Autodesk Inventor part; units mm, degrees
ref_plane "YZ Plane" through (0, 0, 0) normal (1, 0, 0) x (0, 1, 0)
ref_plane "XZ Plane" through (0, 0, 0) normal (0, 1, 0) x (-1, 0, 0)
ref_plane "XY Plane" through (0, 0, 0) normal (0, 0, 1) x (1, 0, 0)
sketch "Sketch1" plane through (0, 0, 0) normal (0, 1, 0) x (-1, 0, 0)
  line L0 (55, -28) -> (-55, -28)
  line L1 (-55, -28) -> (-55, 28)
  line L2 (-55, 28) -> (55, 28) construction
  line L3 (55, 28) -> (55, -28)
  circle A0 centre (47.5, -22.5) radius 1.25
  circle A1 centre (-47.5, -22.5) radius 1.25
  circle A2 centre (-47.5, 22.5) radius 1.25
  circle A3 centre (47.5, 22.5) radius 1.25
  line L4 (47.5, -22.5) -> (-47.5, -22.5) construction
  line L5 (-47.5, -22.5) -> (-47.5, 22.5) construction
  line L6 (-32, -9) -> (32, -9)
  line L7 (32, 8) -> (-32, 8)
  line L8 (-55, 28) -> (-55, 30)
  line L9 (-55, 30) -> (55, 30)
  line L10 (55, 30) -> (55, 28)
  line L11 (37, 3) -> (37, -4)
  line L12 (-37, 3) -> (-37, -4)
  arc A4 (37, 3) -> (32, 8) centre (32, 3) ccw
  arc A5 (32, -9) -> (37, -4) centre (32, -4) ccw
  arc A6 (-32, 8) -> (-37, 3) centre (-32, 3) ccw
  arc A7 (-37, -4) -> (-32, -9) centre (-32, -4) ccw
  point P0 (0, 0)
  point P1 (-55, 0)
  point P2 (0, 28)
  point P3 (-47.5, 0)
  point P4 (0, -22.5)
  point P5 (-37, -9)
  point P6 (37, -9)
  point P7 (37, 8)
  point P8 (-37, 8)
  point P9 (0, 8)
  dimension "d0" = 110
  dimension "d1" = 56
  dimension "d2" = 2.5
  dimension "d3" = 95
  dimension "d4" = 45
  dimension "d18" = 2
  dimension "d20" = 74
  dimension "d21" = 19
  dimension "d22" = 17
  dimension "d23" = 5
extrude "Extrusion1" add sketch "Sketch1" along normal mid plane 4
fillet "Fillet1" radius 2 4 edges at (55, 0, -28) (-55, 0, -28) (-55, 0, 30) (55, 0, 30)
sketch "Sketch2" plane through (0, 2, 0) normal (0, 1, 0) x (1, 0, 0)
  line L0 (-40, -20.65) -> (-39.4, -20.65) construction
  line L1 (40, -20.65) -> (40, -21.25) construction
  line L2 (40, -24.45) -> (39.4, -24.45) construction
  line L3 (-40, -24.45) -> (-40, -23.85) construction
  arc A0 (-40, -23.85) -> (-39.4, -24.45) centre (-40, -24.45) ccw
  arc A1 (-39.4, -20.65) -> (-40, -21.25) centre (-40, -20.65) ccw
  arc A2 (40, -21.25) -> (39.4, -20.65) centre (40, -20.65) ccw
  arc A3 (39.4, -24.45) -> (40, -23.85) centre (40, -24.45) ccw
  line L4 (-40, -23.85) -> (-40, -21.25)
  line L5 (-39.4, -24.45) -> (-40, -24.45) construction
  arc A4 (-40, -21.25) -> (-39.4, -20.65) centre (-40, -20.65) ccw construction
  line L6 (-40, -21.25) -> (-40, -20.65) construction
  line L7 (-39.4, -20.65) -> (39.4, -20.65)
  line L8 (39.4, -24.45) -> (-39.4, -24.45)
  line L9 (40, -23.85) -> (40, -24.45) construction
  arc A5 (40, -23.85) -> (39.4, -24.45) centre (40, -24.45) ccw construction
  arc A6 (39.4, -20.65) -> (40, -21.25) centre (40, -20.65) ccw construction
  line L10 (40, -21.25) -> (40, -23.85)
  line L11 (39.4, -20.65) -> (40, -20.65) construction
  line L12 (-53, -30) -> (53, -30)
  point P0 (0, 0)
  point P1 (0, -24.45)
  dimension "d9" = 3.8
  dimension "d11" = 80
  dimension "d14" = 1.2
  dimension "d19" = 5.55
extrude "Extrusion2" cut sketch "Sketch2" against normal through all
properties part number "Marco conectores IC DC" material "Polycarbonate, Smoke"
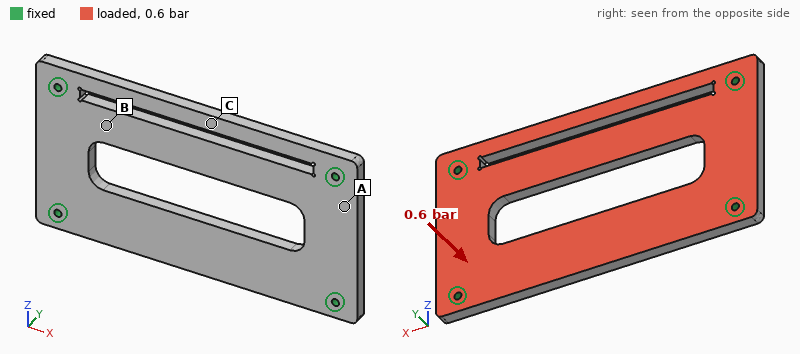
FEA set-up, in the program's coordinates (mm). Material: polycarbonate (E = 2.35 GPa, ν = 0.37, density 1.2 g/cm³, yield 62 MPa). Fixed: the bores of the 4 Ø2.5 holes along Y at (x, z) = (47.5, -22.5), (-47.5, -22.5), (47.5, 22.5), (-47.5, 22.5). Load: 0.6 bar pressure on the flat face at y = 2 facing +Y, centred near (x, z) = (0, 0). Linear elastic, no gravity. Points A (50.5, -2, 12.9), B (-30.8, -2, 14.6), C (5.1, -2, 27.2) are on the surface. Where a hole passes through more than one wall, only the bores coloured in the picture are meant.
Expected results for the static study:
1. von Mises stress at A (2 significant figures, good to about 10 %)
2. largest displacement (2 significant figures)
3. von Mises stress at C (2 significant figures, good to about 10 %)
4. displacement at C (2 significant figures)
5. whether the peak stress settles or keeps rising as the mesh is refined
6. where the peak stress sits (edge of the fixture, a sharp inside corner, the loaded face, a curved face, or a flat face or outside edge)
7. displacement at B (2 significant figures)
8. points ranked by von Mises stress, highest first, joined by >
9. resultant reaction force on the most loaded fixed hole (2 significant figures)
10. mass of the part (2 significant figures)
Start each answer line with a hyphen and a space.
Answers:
- 5.2 MPa
- 1.3 mm
- 8.3 MPa
- 1.0 mm
- keeps rising
- edge of the fixture
- 0.51 mm
- C > A > B
- 73 N
- 23 g
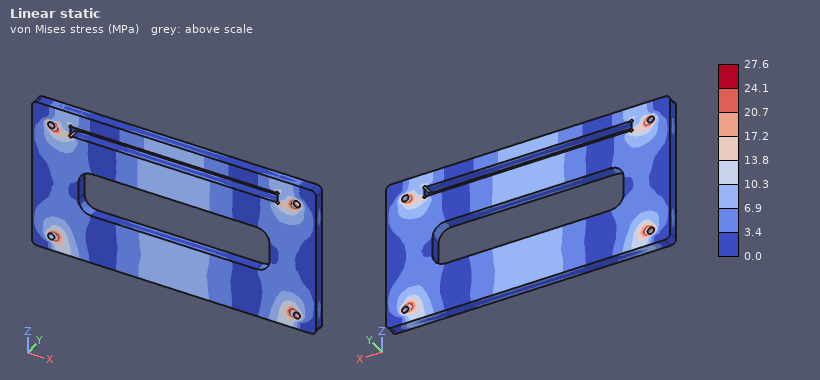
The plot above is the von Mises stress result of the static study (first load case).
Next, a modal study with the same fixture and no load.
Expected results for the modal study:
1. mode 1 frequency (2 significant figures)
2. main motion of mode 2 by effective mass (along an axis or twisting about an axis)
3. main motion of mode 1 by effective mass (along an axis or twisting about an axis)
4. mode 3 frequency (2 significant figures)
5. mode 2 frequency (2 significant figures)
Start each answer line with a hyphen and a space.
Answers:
- 590 Hz
- twisting about X
- along Y
- 680 Hz
- 650 Hz
